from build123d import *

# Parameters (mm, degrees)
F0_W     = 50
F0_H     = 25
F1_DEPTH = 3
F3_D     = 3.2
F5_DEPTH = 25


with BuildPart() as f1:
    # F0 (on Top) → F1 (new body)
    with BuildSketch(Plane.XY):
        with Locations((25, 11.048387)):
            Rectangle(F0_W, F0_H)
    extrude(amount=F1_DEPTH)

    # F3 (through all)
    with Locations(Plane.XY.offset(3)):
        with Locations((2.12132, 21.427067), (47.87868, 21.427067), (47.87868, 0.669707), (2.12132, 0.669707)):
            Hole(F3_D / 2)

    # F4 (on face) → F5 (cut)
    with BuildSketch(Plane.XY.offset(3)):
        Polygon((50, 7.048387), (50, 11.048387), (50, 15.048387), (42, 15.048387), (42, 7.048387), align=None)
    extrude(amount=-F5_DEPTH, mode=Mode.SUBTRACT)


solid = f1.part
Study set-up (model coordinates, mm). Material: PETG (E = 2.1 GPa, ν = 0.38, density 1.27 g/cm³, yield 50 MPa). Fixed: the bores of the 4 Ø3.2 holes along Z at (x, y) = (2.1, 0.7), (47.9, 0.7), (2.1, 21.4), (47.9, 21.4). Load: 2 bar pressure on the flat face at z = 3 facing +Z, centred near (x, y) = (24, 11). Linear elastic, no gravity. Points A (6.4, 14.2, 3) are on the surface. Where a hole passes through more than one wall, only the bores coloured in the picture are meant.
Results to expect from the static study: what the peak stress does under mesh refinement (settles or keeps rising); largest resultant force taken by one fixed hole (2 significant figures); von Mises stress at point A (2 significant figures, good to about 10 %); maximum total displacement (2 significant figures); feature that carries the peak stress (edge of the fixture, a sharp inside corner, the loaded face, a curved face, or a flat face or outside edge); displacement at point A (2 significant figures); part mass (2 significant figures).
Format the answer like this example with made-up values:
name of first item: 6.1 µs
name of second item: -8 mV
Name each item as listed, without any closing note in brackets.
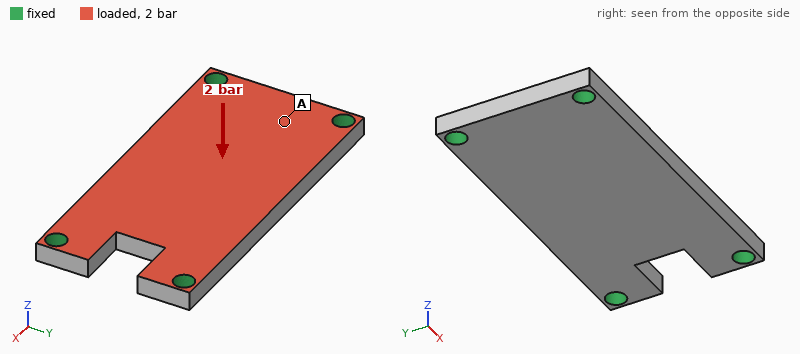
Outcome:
what the peak stress does under mesh refinement: keeps rising
largest resultant force taken by one fixed hole: 61 N
von Mises stress at point A: 5.7 MPa
maximum total displacement: 0.58 mm
feature that carries the peak stress: edge of the fixture
displacement at point A: 0.12 mm
part mass: 4.4 g
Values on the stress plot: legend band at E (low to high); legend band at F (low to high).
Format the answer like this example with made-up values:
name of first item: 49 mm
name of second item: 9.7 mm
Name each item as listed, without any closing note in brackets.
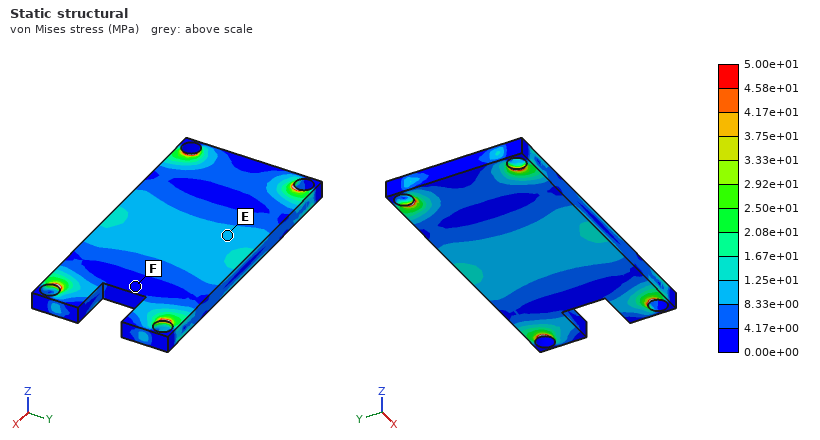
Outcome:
legend band at E: 8.33e+00 to 1.25e+01 MPa
legend band at F: 0.00e+00 to 4.17e+00 MPa
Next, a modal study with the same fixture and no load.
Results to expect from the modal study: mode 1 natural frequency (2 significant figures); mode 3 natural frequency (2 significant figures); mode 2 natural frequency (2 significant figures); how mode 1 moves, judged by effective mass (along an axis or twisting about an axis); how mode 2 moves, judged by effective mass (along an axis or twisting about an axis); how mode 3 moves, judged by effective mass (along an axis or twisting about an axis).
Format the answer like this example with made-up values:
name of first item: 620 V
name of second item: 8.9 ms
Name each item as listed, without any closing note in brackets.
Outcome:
mode 1 natural frequency: 1800 Hz
mode 3 natural frequency: 4700 Hz
mode 2 natural frequency: 2900 Hz
how mode 1 moves, judged by effective mass: along Z
how mode 2 moves, judged by effective mass: twisting about X
how mode 3 moves, judged by effective mass: twisting about Y
